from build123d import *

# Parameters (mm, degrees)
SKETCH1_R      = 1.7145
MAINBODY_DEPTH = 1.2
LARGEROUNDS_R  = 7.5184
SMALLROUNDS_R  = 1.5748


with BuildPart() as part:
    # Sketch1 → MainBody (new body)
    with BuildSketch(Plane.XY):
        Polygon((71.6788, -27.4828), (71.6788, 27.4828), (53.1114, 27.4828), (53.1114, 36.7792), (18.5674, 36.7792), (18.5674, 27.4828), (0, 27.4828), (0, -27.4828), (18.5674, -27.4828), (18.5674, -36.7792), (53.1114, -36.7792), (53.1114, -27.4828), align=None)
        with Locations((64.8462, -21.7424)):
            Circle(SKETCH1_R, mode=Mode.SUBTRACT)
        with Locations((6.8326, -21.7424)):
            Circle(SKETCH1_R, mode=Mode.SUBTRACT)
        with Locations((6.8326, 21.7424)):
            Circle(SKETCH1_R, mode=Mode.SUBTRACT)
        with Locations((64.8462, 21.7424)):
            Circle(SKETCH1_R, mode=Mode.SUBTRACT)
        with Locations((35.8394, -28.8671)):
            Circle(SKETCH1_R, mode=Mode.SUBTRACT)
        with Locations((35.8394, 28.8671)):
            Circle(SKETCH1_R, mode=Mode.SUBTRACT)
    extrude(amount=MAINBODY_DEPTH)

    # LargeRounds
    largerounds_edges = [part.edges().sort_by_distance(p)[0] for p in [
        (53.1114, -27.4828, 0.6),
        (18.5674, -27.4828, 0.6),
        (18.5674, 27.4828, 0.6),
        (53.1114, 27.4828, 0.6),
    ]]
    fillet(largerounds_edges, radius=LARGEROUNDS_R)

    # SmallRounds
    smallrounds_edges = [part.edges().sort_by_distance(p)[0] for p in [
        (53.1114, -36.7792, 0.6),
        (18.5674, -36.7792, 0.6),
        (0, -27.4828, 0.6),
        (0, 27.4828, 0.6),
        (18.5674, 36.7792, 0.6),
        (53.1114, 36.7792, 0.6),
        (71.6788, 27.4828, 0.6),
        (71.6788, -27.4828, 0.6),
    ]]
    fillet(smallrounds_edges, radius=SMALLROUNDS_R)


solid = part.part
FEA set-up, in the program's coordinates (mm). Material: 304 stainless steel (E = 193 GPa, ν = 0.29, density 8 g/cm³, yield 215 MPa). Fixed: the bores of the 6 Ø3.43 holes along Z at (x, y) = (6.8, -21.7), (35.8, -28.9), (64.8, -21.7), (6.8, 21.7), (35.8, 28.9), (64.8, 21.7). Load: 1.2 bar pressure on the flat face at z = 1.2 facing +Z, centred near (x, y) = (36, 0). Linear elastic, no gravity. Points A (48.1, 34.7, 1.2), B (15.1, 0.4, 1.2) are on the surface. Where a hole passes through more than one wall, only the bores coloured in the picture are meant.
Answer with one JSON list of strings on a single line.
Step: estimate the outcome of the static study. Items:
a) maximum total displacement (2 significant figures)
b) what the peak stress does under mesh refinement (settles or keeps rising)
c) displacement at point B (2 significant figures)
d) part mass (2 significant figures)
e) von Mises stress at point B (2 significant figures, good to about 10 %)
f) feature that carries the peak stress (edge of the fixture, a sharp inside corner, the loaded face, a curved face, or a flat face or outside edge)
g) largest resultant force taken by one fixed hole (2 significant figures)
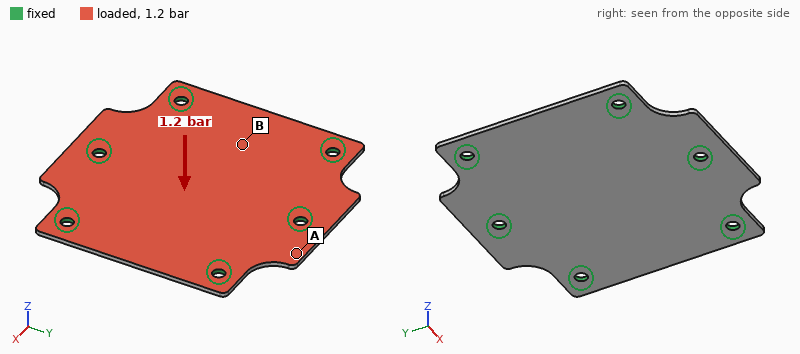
["93 µm", "keeps rising", "65 µm", "44 g", "44 MPa", "edge of the fixture", "110 N"]
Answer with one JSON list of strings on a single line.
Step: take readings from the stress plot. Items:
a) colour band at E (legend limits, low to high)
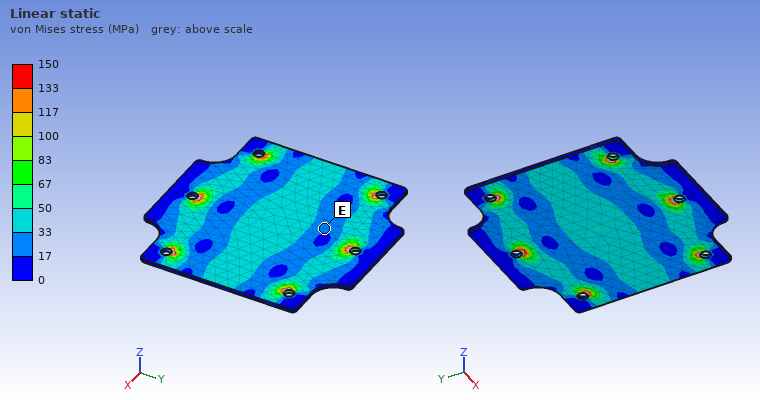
["17 to 33 MPa"]
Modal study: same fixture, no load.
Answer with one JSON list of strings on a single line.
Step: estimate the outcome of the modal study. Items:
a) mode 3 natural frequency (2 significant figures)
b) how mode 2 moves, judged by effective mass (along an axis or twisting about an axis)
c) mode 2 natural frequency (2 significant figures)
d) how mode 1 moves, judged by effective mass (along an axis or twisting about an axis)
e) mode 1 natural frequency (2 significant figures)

["4100 Hz", "twisting about Y", "3300 Hz", "along Z", "2300 Hz"]
